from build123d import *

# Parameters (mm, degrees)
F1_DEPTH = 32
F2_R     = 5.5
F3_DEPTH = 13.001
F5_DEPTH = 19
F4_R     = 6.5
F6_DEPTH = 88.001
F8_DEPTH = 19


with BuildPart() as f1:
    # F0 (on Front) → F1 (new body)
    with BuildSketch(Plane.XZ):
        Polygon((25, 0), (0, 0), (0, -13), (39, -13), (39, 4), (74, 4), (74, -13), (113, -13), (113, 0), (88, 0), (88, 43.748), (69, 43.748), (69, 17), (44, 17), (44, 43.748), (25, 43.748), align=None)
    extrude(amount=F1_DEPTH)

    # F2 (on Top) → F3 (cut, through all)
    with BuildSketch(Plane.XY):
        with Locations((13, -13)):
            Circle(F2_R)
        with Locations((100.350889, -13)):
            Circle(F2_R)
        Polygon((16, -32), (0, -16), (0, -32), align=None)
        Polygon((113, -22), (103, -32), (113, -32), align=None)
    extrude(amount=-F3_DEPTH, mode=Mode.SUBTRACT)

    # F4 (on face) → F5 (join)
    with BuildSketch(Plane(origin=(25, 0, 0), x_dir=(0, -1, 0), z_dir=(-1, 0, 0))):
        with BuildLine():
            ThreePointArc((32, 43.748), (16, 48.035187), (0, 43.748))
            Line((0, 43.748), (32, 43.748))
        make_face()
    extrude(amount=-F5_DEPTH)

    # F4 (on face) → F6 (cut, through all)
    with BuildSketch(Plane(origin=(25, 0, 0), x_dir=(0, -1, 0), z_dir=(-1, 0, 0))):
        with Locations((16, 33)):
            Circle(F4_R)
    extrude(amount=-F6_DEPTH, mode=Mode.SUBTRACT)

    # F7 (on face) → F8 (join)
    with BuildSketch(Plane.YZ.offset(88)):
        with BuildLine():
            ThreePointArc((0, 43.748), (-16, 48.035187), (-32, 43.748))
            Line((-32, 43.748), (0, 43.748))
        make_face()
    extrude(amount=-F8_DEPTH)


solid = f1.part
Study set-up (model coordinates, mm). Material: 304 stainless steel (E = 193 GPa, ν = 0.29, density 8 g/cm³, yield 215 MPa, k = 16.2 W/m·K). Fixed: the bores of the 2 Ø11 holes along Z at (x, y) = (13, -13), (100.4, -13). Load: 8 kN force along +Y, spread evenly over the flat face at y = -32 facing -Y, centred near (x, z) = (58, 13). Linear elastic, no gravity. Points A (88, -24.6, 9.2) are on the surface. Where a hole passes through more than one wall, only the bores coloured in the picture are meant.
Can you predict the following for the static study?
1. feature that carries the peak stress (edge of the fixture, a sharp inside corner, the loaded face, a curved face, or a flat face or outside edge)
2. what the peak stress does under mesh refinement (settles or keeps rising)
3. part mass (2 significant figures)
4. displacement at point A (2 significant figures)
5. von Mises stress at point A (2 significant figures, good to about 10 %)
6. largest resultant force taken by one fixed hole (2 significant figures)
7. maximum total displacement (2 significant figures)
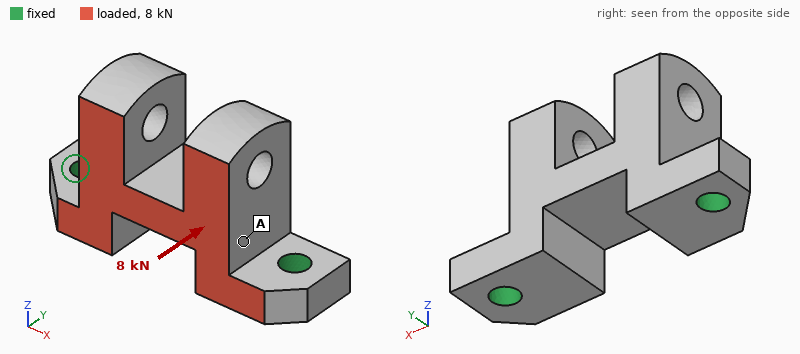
edge of the fixture
keeps rising
710 g
19 µm
23 MPa
4.1 kN
52 µm
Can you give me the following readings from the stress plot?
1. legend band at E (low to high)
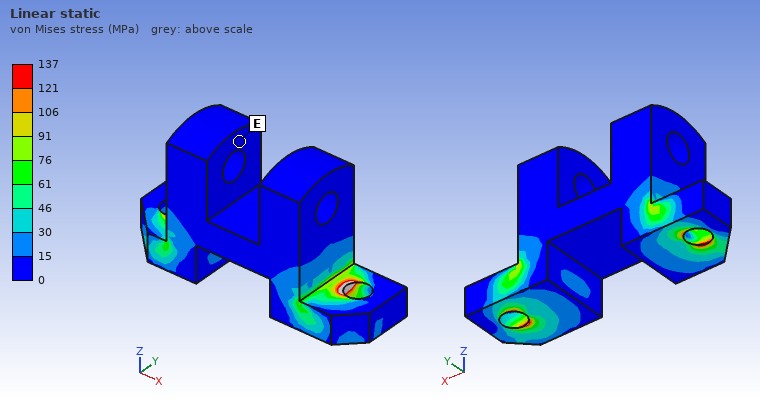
0 to 15 MPa
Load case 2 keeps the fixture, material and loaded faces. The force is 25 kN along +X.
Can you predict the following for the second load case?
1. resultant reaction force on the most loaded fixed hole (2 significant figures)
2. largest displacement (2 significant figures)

15 kN
54 µm
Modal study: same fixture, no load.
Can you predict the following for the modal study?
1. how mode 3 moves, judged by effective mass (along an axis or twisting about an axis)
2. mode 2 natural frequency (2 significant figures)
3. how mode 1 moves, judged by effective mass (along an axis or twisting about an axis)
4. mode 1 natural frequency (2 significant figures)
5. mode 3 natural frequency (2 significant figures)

along X
5000 Hz
along Y
2900 Hz
6200 Hz
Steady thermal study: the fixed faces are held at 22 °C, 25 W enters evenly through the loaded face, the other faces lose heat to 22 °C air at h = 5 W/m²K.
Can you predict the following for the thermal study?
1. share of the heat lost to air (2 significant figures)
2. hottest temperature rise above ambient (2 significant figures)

11 %
54 K
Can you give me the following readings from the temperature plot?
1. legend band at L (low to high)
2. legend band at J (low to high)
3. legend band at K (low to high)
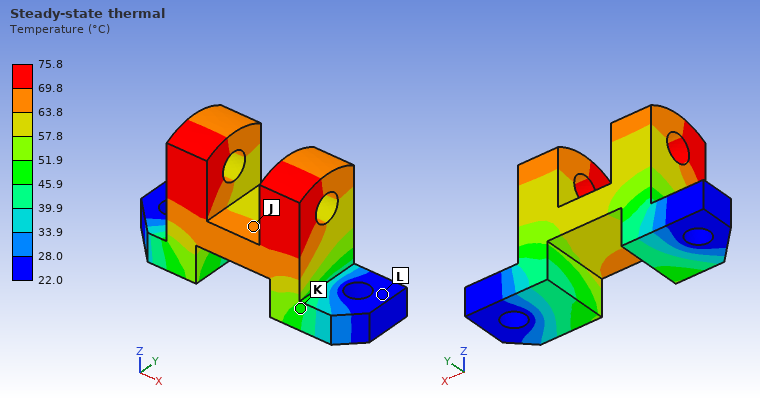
22.0 to 28.0 °C
63.8 to 69.8 °C
45.9 to 51.9 °C
